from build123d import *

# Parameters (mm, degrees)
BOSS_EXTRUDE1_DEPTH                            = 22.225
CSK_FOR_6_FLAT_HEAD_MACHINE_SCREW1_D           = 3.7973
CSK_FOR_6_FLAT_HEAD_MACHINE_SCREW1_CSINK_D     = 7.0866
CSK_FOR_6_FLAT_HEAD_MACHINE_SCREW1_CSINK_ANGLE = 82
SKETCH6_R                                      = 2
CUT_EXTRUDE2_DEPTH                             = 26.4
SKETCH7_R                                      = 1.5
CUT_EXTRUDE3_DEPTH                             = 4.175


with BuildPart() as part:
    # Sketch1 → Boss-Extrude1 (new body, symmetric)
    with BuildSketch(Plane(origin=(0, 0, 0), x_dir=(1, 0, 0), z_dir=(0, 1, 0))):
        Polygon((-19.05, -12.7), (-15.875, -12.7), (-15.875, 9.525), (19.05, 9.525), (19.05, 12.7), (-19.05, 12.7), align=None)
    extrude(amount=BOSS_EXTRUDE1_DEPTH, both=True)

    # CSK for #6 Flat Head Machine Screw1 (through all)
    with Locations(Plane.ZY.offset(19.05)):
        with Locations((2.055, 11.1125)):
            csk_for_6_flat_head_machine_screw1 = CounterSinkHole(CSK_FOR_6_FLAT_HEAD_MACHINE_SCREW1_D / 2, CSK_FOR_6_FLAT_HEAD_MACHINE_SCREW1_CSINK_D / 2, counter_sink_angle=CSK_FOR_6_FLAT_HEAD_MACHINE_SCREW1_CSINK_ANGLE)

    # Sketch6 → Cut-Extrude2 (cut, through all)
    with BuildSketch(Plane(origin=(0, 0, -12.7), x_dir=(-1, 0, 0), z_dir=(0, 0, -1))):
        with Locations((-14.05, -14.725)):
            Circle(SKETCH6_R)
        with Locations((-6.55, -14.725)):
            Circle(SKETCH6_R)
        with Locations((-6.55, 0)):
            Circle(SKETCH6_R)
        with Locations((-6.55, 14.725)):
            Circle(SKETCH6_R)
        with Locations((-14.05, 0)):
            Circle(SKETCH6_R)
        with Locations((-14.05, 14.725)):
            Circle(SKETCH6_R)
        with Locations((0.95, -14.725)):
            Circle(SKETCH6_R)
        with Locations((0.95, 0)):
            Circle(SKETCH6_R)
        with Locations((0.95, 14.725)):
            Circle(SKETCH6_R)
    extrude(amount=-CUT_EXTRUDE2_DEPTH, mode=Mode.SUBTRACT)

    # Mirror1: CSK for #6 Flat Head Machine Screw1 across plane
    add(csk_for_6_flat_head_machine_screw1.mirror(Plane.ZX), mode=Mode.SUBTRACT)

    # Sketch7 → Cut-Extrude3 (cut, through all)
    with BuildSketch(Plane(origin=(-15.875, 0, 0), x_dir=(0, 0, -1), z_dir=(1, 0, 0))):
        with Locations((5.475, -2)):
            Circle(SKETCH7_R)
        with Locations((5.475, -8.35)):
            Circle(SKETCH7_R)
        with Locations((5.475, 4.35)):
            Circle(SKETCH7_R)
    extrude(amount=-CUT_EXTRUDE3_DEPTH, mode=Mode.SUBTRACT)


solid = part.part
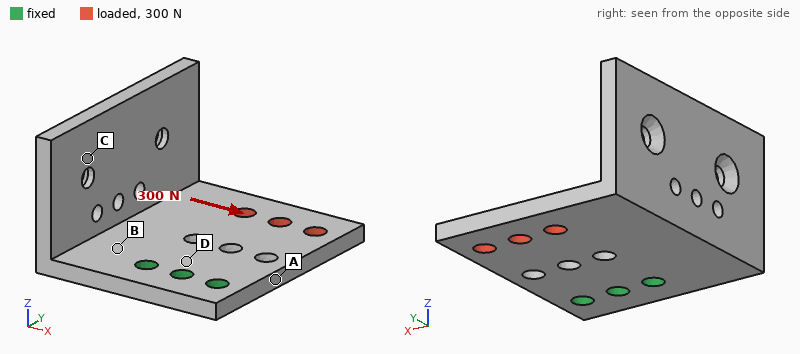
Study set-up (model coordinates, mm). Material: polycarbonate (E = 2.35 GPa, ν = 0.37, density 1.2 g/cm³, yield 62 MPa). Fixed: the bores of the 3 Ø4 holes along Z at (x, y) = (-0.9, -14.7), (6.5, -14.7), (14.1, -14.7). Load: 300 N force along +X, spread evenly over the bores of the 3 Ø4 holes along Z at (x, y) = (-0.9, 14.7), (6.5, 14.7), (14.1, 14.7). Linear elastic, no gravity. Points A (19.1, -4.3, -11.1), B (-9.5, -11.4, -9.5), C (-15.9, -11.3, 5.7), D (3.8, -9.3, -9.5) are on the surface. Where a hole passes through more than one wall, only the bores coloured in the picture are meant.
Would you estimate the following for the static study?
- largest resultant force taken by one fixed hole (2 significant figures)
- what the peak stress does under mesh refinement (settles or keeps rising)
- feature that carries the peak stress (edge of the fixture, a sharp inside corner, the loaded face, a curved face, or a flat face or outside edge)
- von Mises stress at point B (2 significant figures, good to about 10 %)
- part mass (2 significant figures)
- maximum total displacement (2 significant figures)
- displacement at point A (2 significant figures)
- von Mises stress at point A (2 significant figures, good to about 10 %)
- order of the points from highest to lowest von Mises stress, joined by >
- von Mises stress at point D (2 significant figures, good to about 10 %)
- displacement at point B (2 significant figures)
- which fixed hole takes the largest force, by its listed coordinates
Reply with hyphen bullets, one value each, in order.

- 510 N
- keeps rising
- edge of the fixture
- 5.3 MPa
- 9.6 g
- 0.52 mm
- 0.14 mm
- 17 MPa
- A > D > B > C
- 13 MPa
- 0.12 mm
- (-0.9, -14.7)
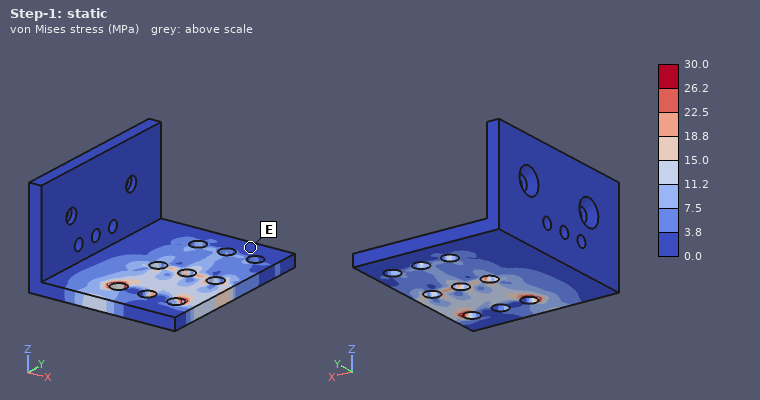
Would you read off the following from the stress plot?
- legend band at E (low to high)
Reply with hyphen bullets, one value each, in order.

- 0.0 to 3.8 MPa
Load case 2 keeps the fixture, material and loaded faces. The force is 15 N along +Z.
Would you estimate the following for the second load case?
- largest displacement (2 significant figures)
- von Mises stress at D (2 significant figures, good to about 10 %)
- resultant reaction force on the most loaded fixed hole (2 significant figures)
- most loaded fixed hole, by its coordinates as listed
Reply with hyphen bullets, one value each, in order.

- 0.68 mm
- 5.3 MPa
- 7.8 N
- (6.5, -14.7)
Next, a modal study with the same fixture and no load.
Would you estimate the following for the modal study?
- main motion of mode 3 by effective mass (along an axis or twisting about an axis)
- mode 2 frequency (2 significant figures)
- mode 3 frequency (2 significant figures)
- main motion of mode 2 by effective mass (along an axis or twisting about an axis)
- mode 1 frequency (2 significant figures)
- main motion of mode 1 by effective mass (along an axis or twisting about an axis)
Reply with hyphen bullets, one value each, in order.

- along Z
- 570 Hz
- 1100 Hz
- along X
- 360 Hz
- along Z
